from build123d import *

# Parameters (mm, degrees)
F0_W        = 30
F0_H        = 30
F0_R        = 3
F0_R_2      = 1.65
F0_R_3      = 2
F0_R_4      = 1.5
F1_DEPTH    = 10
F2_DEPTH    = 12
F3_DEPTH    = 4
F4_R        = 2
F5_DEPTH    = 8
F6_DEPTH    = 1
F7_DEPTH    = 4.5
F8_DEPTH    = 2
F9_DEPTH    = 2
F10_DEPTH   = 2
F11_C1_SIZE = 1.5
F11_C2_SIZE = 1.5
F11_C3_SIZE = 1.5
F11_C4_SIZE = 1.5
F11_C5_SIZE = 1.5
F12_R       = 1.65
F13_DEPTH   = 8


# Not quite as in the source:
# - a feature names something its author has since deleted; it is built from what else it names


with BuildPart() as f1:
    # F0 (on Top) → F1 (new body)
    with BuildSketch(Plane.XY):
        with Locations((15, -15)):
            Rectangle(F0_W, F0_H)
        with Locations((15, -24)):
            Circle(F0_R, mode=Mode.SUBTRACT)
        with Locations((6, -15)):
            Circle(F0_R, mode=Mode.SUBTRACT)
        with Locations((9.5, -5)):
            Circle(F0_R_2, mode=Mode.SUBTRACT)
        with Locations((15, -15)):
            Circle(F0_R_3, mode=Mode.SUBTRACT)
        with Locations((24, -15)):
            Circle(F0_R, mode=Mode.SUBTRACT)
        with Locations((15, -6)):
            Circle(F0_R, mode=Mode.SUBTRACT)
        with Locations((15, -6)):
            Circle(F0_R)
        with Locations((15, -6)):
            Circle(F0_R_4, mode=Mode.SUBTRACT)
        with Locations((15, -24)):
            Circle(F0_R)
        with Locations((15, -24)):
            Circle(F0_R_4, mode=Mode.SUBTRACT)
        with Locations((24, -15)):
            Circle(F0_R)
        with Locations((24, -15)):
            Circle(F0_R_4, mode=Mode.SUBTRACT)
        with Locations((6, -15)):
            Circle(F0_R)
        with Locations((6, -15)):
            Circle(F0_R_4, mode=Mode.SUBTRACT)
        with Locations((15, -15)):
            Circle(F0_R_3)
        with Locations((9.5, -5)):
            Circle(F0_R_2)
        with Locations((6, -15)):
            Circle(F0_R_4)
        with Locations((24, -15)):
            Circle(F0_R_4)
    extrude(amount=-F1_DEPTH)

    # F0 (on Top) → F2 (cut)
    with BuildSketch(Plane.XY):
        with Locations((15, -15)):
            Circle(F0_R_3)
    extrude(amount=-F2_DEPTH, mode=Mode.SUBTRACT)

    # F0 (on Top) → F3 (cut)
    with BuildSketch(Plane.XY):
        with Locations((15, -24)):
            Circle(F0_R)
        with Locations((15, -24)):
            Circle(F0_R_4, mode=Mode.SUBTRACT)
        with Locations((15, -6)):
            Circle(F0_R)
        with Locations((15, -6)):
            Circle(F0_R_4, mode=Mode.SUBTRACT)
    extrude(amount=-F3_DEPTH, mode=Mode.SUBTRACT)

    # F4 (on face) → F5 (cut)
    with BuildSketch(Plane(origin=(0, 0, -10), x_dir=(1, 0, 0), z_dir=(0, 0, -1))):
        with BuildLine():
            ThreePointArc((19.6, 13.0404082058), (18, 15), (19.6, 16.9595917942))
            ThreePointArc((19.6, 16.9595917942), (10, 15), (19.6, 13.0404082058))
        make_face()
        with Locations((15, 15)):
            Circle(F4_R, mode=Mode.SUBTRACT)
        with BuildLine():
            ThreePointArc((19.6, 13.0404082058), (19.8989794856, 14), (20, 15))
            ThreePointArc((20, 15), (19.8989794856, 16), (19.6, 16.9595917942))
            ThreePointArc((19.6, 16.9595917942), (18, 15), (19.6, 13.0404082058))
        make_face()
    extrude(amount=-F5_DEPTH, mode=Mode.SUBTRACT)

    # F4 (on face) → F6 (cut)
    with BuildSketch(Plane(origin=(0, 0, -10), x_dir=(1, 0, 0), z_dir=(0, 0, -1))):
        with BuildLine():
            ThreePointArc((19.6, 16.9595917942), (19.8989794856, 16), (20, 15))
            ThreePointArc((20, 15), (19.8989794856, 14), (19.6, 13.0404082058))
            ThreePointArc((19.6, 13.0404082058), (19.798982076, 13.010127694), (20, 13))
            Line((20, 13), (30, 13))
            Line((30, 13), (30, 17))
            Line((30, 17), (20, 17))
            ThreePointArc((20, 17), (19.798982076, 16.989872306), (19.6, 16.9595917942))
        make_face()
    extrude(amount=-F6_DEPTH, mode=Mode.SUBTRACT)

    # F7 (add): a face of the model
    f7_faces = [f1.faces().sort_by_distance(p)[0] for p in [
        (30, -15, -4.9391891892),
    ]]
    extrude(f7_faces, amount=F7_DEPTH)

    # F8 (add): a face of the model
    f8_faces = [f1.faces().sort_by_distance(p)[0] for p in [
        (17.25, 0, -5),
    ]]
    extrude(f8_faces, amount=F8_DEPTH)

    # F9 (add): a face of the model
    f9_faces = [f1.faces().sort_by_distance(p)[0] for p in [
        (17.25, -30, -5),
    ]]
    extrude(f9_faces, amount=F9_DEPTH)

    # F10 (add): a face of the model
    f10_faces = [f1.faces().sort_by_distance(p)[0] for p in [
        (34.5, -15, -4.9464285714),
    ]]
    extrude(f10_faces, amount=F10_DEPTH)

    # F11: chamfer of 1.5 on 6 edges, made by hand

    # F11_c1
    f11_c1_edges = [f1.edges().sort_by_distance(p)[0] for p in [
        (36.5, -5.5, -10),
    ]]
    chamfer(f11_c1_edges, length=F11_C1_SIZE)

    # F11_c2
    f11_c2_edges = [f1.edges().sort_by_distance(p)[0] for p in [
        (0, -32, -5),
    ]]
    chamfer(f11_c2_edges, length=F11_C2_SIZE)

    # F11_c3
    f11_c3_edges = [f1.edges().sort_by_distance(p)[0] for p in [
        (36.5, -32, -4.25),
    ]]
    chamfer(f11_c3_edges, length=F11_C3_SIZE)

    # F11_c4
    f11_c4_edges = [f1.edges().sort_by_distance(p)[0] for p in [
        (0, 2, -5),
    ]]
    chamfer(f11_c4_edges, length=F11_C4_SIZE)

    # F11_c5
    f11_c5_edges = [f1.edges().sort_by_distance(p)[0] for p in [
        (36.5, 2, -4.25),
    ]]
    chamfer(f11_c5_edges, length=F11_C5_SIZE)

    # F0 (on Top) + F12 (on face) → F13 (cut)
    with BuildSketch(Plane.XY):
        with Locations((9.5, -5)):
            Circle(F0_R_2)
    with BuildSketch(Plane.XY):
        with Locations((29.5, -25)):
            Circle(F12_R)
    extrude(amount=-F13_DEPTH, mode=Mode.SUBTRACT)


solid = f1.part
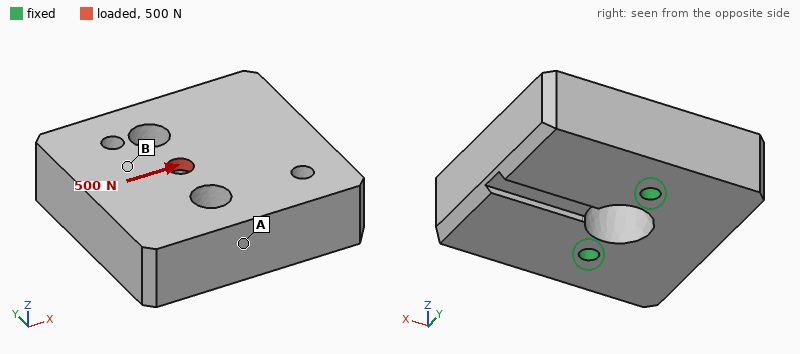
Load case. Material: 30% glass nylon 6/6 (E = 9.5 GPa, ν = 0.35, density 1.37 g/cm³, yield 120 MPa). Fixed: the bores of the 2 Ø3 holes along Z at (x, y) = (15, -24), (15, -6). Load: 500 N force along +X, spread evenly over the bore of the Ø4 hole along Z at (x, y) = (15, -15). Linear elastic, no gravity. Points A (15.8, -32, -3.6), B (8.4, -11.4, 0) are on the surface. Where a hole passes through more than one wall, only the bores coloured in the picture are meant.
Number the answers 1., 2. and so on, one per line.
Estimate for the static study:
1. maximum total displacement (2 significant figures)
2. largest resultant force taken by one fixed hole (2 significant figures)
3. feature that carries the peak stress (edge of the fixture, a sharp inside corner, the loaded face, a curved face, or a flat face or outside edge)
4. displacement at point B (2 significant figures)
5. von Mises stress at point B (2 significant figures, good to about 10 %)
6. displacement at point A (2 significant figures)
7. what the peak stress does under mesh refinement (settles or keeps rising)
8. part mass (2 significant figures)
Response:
1. 43 µm
2. 250 N
3. edge of the fixture
4. 21 µm
5. 6.4 MPa
6. 6.7 µm
7. keeps rising
8. 15 g
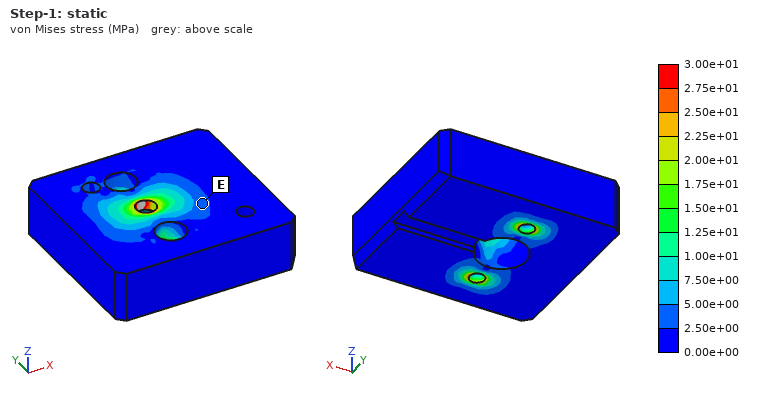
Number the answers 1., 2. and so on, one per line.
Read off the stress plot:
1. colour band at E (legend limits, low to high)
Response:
1. 2.50e+00 to 5.00e+00 MPa
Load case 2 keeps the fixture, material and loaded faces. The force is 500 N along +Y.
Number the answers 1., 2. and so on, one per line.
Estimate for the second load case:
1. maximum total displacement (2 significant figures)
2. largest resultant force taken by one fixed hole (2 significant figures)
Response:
1. 19 µm
2. 280 N
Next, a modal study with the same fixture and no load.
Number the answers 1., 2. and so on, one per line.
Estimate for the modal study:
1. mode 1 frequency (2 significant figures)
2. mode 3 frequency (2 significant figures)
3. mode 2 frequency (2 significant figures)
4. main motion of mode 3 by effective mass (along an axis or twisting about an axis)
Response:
1. 4300 Hz
2. 9900 Hz
3. 8900 Hz
4. along Y
